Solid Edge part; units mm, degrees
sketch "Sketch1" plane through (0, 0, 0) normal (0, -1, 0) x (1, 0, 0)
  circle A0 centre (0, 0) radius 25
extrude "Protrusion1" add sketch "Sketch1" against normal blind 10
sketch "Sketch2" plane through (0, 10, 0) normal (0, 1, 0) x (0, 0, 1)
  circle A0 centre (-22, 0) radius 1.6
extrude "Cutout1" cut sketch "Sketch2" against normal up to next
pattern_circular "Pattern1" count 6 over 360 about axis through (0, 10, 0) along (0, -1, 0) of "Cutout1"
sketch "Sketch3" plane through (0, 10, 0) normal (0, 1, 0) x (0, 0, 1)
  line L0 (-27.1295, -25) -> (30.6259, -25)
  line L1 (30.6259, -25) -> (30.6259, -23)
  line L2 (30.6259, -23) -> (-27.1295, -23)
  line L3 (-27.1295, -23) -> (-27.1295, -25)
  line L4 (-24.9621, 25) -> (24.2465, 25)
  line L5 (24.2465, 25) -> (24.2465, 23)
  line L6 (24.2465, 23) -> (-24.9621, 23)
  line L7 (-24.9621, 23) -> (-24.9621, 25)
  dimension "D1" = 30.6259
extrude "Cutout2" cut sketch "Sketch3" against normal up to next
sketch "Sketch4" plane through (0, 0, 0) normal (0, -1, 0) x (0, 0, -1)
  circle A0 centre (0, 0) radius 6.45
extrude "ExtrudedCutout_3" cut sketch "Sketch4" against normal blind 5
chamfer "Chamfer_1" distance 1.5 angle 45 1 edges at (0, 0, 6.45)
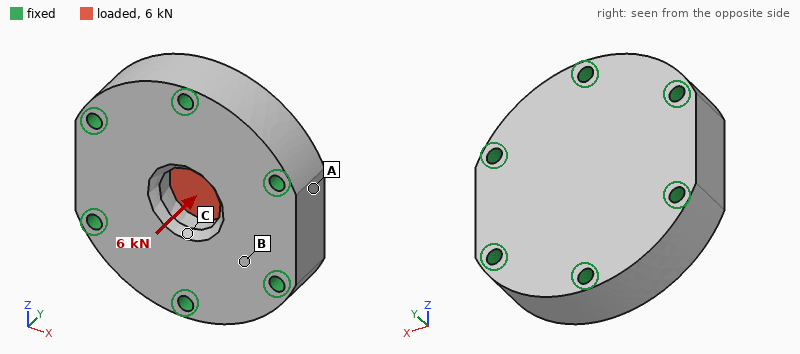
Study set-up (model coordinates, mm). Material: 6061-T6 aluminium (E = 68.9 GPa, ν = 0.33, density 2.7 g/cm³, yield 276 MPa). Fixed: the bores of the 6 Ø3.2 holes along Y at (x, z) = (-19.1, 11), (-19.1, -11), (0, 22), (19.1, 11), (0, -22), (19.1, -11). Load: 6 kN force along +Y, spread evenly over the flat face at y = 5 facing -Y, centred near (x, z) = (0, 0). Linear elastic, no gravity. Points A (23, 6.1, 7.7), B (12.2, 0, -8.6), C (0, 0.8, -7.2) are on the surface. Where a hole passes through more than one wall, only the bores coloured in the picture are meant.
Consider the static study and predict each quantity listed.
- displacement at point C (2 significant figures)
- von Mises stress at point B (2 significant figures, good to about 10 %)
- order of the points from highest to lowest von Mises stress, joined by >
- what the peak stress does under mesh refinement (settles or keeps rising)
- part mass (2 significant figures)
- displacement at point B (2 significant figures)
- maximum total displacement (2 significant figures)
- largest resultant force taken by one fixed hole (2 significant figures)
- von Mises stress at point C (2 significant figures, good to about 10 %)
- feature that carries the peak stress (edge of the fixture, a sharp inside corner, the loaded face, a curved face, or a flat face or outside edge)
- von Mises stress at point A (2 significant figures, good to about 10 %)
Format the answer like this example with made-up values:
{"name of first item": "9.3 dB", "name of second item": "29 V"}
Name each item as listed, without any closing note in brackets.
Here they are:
{"displacement at point C": "16 µm", "von Mises stress at point B": "30 MPa", "order of the points from highest to lowest von Mises stress, joined by >": "C > B > A", "what the peak stress does under mesh refinement": "keeps rising", "part mass": "48 g", "displacement at point B": "7.3 µm", "maximum total displacement": "28 µm", "largest resultant force taken by one fixed hole": "1.1 kN", "von Mises stress at point C": "48 MPa", "feature that carries the peak stress": "edge of the fixture", "von Mises stress at point A": "12 MPa"}
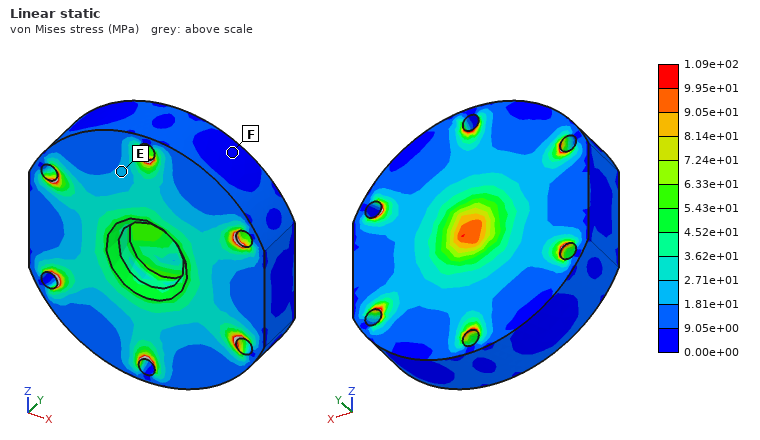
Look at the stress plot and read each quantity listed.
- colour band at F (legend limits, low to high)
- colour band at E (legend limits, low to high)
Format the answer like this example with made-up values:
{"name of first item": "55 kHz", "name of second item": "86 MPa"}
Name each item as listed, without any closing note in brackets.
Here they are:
{"colour band at F": "0.00e+00 to 9.05e+00 MPa", "colour band at E": "1.81e+01 to 2.71e+01 MPa"}
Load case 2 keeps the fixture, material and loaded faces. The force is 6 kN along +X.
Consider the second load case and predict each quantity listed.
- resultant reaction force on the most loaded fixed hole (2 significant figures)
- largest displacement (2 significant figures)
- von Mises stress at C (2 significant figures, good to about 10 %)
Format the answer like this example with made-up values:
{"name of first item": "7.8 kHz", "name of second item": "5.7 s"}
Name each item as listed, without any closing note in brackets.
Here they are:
{"resultant reaction force on the most loaded fixed hole": "1.4 kN", "largest displacement": "11 µm", "von Mises stress at C": "14 MPa"}
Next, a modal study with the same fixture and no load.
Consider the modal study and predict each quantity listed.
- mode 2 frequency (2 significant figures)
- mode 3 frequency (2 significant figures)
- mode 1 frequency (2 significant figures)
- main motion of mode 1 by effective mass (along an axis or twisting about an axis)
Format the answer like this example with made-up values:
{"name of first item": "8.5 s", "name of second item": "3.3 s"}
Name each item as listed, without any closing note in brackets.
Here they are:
{"mode 2 frequency": "47 kHz", "mode 3 frequency": "48 kHz", "mode 1 frequency": "30 kHz", "main motion of mode 1 by effective mass": "along Y"}
